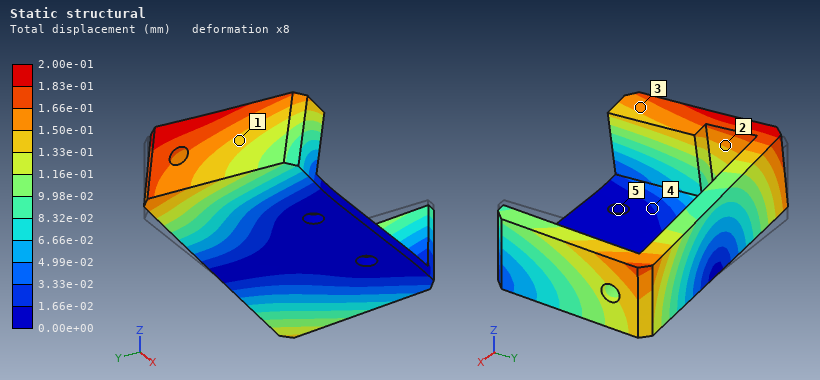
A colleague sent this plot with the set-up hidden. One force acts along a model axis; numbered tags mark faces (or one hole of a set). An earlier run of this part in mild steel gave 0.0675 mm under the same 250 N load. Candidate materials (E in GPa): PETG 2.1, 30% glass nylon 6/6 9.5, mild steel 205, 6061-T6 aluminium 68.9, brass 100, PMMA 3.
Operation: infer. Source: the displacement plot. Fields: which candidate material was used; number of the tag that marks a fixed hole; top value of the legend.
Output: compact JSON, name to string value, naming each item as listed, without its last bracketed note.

{"which candidate material was used": "6061-T6 aluminium", "number of the tag that marks a fixed hole": "5", "top value of the legend": "2.00e-01 mm"}
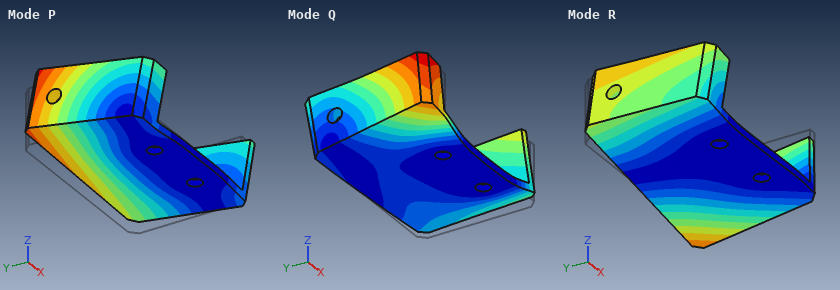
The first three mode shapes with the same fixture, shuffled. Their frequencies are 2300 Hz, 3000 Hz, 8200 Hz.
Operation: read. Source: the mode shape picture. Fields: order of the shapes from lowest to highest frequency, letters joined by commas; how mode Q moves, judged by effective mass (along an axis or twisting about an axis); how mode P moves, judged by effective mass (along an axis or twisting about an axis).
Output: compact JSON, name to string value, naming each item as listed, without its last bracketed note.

{"order of the shapes from lowest to highest frequency, letters joined by commas": "P, R, Q", "how mode Q moves, judged by effective mass": "along Z", "how mode P moves, judged by effective mass": "along Z"}
